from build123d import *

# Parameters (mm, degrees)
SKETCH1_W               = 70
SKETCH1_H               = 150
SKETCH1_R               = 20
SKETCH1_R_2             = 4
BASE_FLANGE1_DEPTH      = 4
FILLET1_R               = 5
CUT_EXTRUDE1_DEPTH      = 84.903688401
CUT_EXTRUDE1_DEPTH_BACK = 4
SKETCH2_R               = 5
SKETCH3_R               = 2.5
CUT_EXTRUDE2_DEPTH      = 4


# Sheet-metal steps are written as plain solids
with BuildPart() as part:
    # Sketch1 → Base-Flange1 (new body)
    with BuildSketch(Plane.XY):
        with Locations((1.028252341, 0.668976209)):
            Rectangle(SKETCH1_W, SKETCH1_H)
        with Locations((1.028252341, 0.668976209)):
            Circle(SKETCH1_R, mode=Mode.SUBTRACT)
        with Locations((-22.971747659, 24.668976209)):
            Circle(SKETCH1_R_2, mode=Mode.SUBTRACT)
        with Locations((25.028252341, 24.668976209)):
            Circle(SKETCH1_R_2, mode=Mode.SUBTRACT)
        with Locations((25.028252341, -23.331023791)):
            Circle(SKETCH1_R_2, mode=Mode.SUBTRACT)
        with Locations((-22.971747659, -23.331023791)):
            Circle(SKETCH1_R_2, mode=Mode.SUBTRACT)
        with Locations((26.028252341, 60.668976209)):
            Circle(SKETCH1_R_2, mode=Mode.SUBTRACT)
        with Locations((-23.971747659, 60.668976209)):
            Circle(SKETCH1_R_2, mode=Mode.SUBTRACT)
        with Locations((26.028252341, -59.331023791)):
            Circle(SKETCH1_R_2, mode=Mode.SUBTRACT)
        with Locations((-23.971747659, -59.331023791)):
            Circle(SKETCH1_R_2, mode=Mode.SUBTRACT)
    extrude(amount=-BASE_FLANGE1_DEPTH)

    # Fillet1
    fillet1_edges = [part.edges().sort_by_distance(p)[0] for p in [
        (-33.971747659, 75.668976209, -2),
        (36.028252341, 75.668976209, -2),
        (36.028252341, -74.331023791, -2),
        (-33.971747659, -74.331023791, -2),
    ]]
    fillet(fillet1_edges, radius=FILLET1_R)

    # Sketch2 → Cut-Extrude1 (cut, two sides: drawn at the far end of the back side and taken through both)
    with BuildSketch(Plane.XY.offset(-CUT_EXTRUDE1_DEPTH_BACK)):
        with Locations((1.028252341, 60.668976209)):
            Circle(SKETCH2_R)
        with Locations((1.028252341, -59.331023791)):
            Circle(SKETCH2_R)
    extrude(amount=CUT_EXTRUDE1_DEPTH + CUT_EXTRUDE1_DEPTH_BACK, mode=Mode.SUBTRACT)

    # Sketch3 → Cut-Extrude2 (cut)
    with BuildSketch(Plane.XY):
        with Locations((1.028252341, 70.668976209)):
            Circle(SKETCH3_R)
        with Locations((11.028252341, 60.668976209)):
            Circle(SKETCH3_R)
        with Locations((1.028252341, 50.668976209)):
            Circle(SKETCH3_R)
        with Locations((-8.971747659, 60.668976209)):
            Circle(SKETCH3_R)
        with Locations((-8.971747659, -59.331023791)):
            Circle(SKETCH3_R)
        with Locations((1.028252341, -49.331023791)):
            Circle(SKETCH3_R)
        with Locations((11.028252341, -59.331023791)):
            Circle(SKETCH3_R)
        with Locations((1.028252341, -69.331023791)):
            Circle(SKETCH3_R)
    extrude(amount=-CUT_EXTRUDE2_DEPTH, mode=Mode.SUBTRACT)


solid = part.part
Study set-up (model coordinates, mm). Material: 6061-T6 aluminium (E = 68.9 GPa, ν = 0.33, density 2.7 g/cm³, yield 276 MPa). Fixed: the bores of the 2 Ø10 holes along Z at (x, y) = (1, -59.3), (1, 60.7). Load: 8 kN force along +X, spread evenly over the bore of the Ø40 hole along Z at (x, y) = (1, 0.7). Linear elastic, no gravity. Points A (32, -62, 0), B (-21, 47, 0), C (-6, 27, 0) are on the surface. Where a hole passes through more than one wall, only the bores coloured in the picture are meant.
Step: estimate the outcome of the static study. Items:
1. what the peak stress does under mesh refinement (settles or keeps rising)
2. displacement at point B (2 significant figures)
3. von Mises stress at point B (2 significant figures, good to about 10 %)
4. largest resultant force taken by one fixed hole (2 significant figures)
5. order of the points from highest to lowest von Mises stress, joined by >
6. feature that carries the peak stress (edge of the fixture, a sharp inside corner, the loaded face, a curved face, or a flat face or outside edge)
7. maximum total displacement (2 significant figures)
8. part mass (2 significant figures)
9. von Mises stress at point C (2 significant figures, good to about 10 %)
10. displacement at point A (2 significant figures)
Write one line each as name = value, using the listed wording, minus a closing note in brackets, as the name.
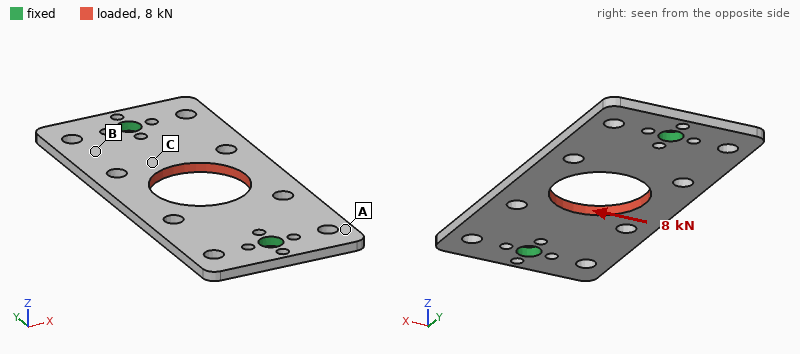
what the peak stress does under mesh refinement = keeps rising
displacement at point B = 29 µm
von Mises stress at point B = 24 MPa
largest resultant force taken by one fixed hole = 4.0 kN
order of the points from highest to lowest von Mises stress, joined by > = C > B > A
feature that carries the peak stress = edge of the fixture
maximum total displacement = 75 µm
part mass = 92 g
von Mises stress at point C = 39 MPa
displacement at point A = 27 µm
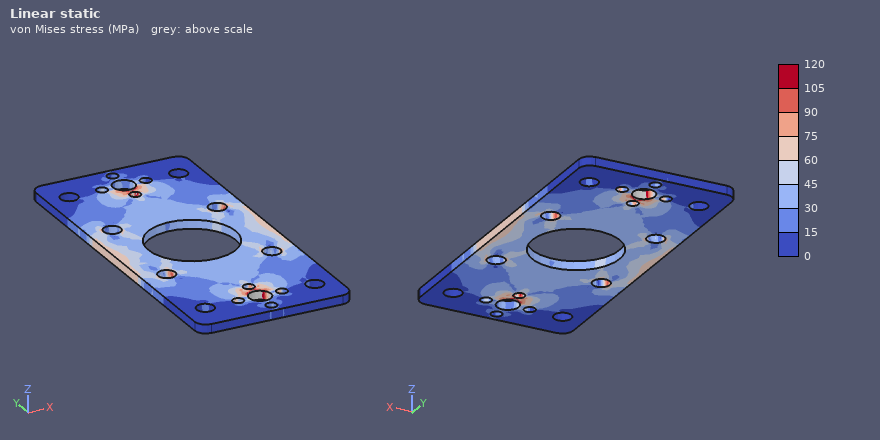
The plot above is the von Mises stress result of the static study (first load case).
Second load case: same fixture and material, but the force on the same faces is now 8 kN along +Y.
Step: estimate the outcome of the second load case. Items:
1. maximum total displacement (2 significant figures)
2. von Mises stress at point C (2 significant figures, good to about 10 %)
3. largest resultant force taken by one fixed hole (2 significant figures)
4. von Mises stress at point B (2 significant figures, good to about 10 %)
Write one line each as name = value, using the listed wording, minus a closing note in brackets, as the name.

maximum total displacement = 25 µm
von Mises stress at point C = 22 MPa
largest resultant force taken by one fixed hole = 4.0 kN
von Mises stress at point B = 10 MPa
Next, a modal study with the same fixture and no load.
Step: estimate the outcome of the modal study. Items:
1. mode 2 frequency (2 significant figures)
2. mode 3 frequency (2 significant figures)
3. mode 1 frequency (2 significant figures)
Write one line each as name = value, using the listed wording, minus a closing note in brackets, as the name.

mode 2 frequency = 1400 Hz
mode 3 frequency = 2600 Hz
mode 1 frequency = 1300 Hz
